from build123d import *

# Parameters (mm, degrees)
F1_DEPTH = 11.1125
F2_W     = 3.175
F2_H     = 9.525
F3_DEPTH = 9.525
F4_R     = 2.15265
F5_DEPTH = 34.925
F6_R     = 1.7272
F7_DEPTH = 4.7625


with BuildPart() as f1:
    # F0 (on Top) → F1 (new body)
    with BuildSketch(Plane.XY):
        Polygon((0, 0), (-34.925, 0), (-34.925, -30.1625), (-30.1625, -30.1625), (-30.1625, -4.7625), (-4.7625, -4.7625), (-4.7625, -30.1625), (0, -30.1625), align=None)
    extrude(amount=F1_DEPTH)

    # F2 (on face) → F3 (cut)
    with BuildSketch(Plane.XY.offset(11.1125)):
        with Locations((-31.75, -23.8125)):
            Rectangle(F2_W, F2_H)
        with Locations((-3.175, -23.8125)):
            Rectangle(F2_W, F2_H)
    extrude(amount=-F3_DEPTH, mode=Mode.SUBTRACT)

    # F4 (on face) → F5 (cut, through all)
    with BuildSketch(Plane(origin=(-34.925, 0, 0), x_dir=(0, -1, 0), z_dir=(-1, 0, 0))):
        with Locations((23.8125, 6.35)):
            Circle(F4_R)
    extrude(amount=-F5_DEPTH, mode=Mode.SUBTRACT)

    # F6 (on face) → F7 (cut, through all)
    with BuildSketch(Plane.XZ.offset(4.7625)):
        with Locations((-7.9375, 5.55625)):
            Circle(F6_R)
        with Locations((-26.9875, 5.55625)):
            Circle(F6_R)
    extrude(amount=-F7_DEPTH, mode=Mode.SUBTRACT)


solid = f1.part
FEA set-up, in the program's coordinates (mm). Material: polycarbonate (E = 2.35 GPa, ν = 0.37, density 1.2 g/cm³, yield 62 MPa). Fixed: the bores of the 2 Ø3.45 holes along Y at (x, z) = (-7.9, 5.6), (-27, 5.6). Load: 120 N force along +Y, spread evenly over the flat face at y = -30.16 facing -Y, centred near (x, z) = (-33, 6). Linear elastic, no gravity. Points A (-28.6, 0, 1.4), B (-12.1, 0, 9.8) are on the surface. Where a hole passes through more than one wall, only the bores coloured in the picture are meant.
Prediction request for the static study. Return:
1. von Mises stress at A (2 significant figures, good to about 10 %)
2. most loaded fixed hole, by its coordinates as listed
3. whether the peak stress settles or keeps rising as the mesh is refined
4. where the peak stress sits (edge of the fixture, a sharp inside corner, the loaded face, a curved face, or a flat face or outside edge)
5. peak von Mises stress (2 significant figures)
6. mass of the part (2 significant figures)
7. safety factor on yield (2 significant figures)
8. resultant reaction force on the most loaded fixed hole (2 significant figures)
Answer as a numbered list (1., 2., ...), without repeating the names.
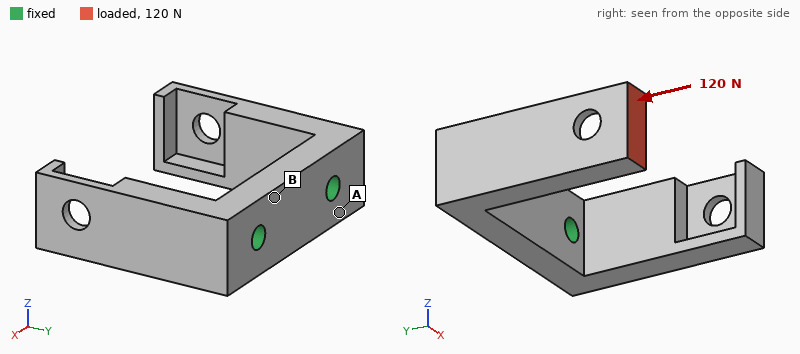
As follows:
1. 5.3 MPa
2. (-27, 5.6)
3. settles
4. a curved face
5. 53 MPa
6. 4.6 g
7. 1.2
8. 120 N
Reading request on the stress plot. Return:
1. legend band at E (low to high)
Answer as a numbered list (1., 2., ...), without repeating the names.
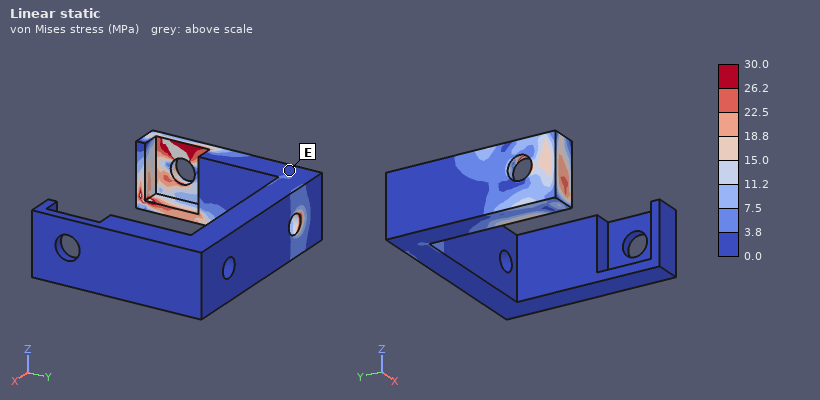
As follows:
1. 0.0 to 3.8 MPa
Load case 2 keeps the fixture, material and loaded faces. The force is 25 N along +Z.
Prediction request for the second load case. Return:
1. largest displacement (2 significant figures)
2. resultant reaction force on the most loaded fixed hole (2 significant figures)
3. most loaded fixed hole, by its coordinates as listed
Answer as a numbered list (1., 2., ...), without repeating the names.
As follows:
1. 0.57 mm
2. 28 N
3. (-27, 5.6)
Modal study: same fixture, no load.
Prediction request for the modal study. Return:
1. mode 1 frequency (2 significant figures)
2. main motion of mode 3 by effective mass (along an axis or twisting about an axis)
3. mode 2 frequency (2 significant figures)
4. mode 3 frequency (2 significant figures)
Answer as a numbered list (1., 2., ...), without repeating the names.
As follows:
1. 1400 Hz
2. along Z
3. 1400 Hz
4. 2100 Hz
